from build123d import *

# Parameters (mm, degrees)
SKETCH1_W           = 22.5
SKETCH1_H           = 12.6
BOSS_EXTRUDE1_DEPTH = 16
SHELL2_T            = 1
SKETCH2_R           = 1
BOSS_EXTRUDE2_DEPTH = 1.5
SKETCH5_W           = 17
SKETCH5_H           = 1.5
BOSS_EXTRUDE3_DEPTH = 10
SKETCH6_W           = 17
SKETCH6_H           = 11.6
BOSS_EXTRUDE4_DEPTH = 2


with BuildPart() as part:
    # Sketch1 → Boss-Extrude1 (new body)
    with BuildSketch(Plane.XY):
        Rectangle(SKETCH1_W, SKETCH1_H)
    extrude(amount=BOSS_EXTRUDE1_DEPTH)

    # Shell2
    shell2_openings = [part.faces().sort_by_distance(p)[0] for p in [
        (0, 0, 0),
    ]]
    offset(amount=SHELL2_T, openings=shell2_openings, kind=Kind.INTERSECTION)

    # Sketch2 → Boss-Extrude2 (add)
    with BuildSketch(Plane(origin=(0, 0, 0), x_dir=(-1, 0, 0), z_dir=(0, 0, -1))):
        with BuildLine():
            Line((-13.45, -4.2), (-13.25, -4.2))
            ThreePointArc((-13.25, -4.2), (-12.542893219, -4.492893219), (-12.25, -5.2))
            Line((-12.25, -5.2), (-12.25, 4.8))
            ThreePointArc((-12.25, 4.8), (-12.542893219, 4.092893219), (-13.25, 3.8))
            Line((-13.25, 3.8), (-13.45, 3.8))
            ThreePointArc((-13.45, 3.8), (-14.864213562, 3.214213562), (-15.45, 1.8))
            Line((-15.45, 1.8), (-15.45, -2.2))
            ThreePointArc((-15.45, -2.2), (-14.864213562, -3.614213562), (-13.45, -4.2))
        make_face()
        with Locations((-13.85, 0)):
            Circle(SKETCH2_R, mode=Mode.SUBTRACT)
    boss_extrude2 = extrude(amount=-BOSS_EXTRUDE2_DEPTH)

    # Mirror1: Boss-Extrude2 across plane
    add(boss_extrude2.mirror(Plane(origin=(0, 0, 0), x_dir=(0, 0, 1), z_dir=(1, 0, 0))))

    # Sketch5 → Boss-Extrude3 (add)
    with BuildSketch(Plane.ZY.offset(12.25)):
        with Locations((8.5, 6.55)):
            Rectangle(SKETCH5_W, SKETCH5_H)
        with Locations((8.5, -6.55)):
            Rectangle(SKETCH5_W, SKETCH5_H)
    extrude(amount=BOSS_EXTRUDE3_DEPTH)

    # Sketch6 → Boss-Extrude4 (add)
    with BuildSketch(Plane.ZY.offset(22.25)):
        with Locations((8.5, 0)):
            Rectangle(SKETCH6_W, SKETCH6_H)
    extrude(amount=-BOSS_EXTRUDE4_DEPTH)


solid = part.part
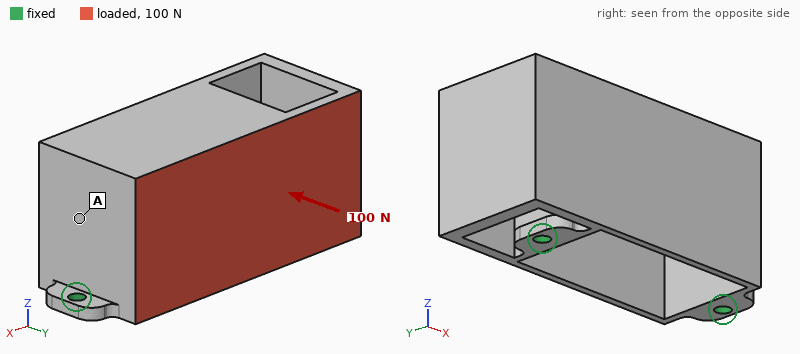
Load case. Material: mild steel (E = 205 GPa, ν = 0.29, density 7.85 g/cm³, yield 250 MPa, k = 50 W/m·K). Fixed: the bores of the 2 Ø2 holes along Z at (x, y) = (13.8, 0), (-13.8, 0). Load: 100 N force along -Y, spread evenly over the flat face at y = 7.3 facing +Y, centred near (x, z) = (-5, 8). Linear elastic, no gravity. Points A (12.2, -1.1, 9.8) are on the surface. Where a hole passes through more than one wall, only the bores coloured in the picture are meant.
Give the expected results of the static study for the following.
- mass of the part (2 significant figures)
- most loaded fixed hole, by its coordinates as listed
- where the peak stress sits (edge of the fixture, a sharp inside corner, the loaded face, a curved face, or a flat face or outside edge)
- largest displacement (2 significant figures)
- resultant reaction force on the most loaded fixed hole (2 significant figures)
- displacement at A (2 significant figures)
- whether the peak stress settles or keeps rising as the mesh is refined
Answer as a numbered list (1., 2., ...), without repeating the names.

1. 20 g
2. (-13.8, 0)
3. edge of the fixture
4. 20 µm
5. 67 N
6. 8.5 µm
7. keeps rising
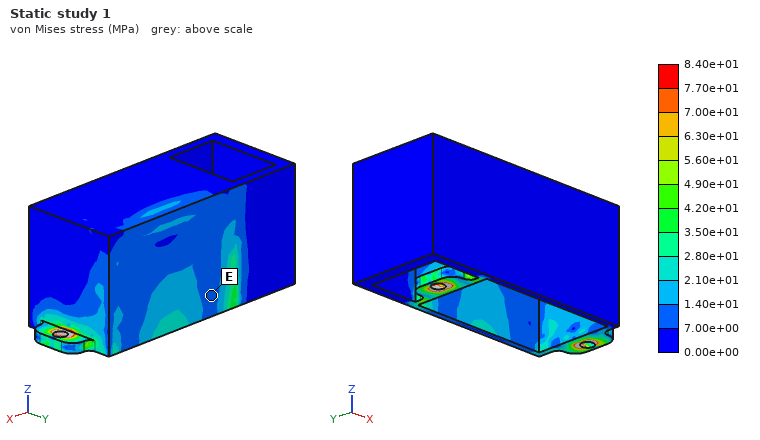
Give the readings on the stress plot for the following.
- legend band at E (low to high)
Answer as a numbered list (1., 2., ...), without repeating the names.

1. 7.00e+00 to 1.40e+01 MPa
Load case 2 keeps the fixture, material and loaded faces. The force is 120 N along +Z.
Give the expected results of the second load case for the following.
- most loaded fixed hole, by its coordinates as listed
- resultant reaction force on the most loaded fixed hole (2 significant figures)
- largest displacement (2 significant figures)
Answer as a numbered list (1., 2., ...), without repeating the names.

1. (-13.8, 0)
2. 85 N
3. 21 µm
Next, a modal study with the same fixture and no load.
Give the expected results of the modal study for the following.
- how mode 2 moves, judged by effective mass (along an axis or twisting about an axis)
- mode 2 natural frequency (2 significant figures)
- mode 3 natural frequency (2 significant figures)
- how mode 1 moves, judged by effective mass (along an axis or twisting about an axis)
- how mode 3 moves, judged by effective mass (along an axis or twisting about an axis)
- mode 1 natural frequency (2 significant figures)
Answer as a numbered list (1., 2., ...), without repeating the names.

1. twisting about Z
2. 5900 Hz
3. 7400 Hz
4. along Y
5. along X
6. 2700 Hz
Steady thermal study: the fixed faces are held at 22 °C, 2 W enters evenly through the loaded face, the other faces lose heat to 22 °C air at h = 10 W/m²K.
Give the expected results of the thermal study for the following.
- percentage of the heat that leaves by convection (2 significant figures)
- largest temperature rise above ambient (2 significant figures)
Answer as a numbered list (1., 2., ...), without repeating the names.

1. 18 %
2. 15 K
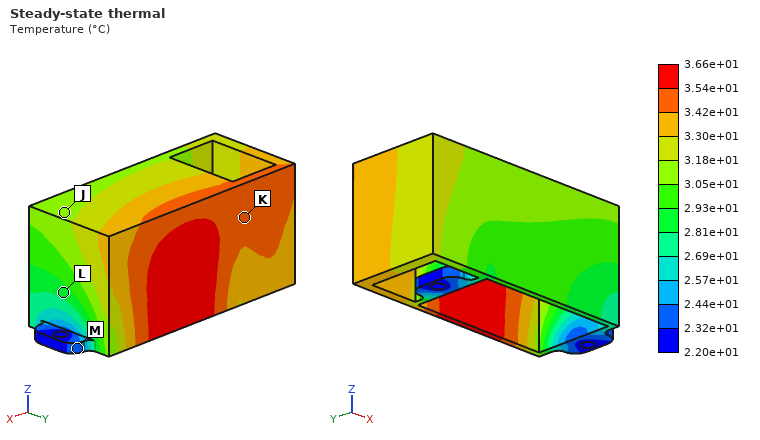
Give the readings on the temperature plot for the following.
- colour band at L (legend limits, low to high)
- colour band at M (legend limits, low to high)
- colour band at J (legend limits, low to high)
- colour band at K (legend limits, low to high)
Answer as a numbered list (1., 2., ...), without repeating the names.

1. 2.81e+01 to 2.93e+01 °C
2. 2.32e+01 to 2.44e+01 °C
3. 3.05e+01 to 3.18e+01 °C
4. 3.42e+01 to 3.54e+01 °C
